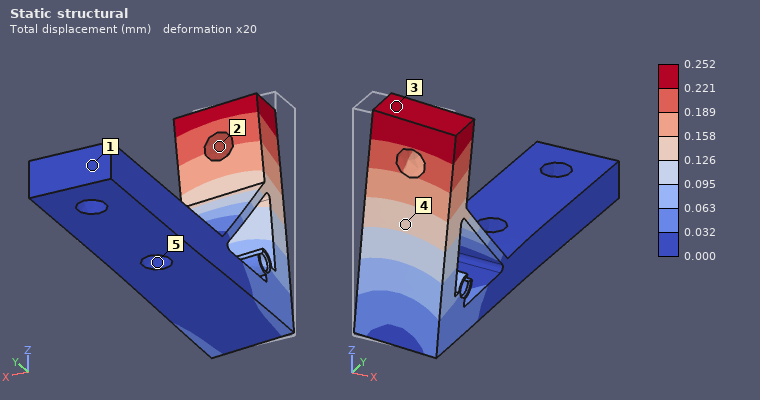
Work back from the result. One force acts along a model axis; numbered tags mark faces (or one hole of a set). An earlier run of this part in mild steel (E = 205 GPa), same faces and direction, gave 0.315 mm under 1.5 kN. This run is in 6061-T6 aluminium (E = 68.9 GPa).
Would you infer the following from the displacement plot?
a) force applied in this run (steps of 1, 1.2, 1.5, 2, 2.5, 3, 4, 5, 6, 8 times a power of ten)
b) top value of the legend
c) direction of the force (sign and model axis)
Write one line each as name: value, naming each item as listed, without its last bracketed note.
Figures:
force applied in this run: 400 N
top value of the legend: 0.252 mm
direction of the force: +X
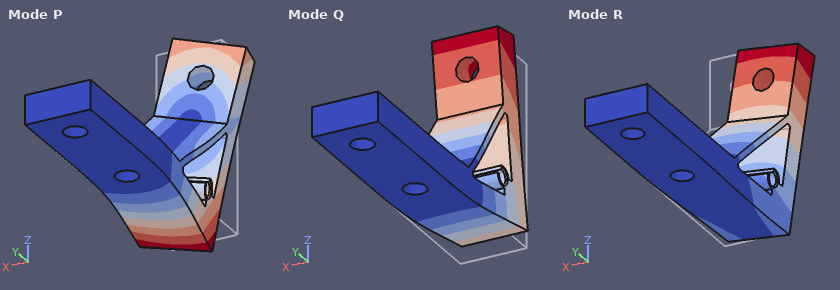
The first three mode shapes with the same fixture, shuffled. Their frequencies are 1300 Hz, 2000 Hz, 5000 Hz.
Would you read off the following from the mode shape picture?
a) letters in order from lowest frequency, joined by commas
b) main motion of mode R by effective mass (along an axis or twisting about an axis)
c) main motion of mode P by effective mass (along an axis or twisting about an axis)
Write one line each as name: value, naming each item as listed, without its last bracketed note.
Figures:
letters in order from lowest frequency, joined by commas: Q, R, P
main motion of mode R by effective mass: along X
main motion of mode P by effective mass: along X
